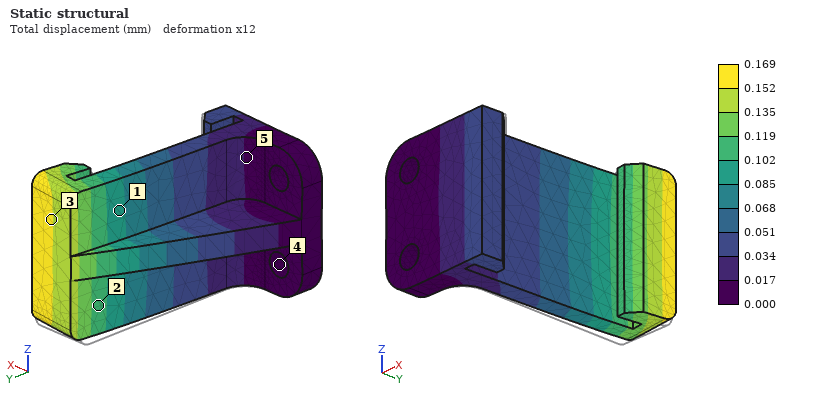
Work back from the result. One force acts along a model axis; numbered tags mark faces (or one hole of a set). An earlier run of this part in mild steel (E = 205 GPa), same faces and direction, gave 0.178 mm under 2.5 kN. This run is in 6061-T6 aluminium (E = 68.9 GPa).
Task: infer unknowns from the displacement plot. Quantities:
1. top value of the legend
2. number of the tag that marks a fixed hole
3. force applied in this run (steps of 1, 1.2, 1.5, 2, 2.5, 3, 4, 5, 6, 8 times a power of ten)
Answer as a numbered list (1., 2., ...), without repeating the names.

1. 0.169 mm
2. 4
3. 800 N
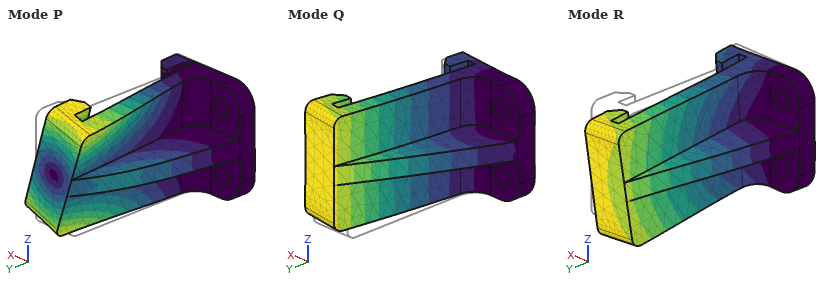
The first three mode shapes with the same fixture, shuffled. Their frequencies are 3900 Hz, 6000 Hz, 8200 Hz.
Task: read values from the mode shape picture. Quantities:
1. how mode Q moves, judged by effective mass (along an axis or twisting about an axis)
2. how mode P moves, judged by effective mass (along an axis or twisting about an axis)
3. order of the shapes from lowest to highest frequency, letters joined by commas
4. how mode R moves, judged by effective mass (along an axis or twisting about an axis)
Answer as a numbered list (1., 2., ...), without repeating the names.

1. along X
2. twisting about Y
3. Q, R, P
4. along Z
